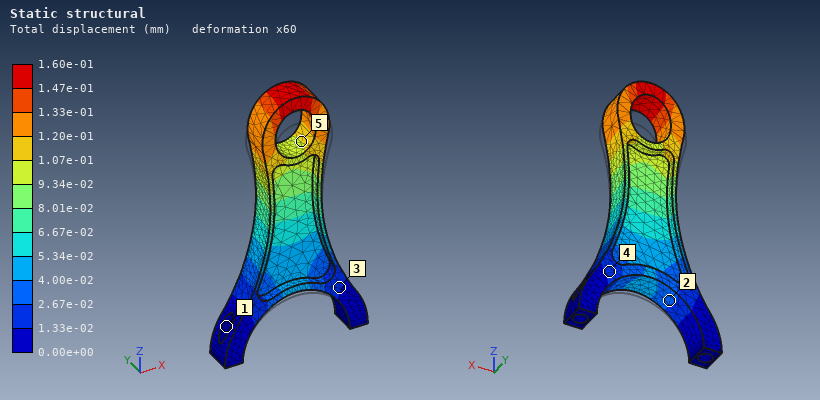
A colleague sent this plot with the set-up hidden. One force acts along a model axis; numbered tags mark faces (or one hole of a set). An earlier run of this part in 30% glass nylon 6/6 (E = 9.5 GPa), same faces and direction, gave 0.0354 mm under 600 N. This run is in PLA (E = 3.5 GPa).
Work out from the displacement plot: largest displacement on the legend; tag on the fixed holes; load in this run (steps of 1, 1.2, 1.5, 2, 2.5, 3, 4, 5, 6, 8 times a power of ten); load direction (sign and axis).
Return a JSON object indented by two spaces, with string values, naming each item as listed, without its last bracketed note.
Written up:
{
  "largest displacement on the legend": "1.60e-01 mm",
  "tag on the fixed holes": "1",
  "load in this run": "1 kN",
  "load direction": "+Z"
}
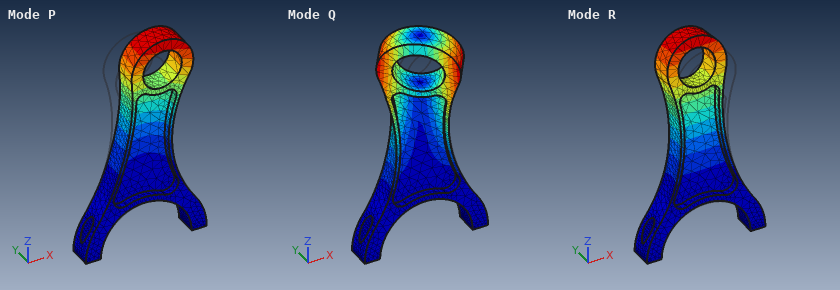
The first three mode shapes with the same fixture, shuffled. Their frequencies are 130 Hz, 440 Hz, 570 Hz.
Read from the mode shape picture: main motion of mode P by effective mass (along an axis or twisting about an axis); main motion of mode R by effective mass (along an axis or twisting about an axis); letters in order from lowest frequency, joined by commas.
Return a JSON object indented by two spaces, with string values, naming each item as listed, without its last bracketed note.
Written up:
{
  "main motion of mode P by effective mass": "along X",
  "main motion of mode R by effective mass": "along Y",
  "letters in order from lowest frequency, joined by commas": "R, Q, P"
}
